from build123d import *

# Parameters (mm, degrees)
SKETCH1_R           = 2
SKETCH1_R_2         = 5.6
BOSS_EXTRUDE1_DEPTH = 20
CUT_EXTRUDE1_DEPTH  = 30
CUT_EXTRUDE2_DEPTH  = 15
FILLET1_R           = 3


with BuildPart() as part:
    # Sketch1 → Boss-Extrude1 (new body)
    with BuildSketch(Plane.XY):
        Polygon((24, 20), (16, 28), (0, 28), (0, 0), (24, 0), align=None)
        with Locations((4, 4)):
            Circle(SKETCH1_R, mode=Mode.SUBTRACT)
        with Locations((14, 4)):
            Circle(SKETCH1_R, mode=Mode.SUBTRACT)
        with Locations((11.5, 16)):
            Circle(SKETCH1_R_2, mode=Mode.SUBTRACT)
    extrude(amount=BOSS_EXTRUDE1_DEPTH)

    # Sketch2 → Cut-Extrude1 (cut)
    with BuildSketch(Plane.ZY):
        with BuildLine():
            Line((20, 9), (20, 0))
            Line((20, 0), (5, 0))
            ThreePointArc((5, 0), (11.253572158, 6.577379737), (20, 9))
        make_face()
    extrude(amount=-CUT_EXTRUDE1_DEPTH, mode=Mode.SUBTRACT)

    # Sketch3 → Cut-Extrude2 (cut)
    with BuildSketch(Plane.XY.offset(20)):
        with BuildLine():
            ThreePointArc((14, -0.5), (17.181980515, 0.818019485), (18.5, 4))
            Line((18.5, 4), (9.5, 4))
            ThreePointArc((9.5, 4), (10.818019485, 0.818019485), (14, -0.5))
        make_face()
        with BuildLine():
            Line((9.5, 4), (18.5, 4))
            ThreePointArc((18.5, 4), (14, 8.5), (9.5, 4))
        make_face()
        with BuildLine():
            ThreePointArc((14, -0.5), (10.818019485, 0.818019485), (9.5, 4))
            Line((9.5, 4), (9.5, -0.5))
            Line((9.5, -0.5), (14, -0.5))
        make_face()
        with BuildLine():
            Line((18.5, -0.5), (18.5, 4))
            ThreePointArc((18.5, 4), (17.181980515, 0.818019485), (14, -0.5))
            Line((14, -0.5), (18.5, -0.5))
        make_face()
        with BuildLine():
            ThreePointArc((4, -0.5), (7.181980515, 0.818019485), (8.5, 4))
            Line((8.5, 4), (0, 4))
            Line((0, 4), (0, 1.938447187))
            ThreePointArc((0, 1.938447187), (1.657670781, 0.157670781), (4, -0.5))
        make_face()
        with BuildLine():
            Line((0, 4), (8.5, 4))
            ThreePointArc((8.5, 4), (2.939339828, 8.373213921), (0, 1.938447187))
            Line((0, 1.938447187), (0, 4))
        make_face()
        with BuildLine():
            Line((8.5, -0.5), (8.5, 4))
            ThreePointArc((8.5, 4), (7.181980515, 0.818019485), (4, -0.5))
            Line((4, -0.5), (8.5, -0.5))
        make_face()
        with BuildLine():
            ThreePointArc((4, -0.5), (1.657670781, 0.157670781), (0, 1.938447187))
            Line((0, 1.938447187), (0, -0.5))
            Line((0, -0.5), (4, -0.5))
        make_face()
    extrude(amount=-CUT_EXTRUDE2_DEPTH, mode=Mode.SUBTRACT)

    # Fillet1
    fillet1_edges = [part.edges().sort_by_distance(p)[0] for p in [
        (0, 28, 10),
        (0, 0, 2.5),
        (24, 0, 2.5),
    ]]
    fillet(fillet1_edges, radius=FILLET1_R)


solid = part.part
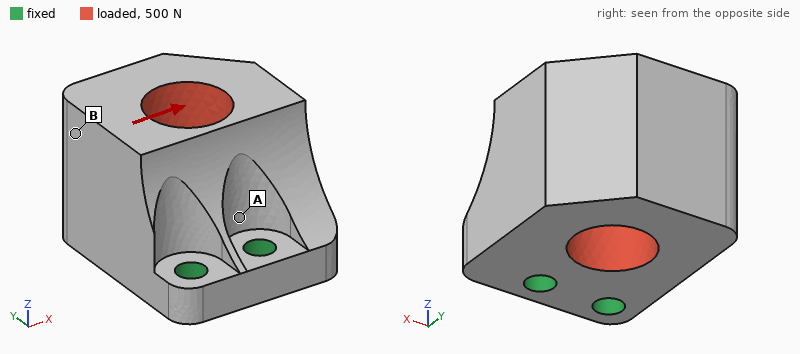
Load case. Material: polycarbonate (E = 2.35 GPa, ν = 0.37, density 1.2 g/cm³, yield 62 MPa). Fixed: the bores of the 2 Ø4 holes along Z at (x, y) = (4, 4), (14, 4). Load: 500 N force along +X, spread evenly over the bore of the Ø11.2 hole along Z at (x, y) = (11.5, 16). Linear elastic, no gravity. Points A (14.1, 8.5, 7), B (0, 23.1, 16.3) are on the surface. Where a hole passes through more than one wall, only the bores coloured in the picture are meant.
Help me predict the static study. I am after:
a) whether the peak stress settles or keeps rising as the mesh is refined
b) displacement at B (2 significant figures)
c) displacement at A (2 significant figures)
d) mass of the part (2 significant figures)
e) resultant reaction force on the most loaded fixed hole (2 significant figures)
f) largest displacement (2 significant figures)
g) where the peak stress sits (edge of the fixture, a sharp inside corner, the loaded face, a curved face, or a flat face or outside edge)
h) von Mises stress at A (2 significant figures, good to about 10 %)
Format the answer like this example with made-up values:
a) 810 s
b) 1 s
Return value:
a) keeps rising
b) 0.29 mm
c) 0.085 mm
d) 9.5 g
e) 540 N
f) 0.35 mm
g) a sharp inside corner
h) 12 MPa
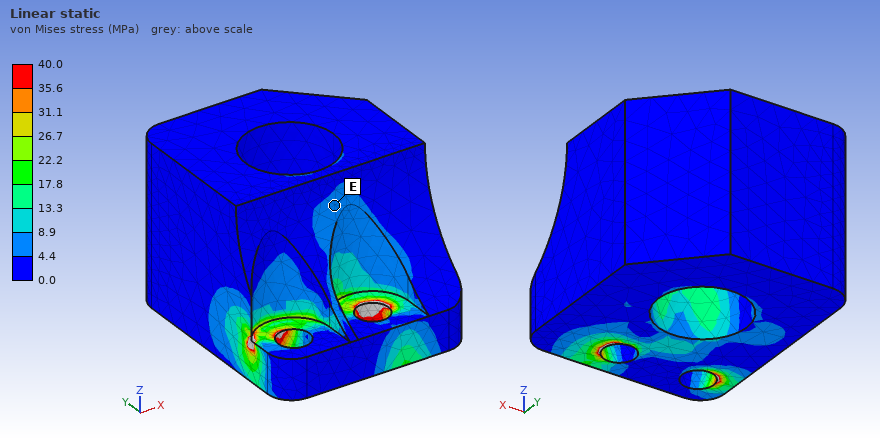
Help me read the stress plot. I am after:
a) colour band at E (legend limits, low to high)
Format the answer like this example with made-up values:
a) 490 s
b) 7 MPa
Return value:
a) 4.4 to 8.9 MPa
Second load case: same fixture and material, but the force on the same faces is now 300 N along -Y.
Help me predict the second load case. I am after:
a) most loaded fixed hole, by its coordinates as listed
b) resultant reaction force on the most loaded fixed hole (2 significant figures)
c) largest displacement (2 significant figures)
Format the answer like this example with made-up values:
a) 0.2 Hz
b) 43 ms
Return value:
a) (14, 4)
b) 200 N
c) 0.48 mm
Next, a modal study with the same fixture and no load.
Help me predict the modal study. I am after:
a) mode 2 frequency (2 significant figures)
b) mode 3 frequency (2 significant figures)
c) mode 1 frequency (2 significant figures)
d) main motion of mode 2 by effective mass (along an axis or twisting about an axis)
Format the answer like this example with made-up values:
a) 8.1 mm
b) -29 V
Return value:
a) 2400 Hz
b) 3200 Hz
c) 1200 Hz
d) along X
